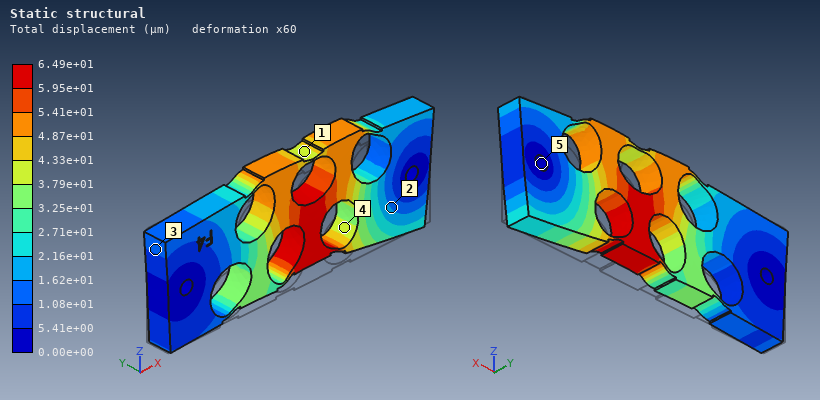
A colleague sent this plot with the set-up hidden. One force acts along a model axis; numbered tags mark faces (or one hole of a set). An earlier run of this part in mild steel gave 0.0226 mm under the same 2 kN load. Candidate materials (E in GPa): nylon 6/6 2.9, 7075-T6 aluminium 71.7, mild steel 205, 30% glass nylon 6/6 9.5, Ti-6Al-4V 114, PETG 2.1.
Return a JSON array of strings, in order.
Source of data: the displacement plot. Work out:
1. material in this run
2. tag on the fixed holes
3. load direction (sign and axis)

["7075-T6 aluminium", "5", "+Z"]
